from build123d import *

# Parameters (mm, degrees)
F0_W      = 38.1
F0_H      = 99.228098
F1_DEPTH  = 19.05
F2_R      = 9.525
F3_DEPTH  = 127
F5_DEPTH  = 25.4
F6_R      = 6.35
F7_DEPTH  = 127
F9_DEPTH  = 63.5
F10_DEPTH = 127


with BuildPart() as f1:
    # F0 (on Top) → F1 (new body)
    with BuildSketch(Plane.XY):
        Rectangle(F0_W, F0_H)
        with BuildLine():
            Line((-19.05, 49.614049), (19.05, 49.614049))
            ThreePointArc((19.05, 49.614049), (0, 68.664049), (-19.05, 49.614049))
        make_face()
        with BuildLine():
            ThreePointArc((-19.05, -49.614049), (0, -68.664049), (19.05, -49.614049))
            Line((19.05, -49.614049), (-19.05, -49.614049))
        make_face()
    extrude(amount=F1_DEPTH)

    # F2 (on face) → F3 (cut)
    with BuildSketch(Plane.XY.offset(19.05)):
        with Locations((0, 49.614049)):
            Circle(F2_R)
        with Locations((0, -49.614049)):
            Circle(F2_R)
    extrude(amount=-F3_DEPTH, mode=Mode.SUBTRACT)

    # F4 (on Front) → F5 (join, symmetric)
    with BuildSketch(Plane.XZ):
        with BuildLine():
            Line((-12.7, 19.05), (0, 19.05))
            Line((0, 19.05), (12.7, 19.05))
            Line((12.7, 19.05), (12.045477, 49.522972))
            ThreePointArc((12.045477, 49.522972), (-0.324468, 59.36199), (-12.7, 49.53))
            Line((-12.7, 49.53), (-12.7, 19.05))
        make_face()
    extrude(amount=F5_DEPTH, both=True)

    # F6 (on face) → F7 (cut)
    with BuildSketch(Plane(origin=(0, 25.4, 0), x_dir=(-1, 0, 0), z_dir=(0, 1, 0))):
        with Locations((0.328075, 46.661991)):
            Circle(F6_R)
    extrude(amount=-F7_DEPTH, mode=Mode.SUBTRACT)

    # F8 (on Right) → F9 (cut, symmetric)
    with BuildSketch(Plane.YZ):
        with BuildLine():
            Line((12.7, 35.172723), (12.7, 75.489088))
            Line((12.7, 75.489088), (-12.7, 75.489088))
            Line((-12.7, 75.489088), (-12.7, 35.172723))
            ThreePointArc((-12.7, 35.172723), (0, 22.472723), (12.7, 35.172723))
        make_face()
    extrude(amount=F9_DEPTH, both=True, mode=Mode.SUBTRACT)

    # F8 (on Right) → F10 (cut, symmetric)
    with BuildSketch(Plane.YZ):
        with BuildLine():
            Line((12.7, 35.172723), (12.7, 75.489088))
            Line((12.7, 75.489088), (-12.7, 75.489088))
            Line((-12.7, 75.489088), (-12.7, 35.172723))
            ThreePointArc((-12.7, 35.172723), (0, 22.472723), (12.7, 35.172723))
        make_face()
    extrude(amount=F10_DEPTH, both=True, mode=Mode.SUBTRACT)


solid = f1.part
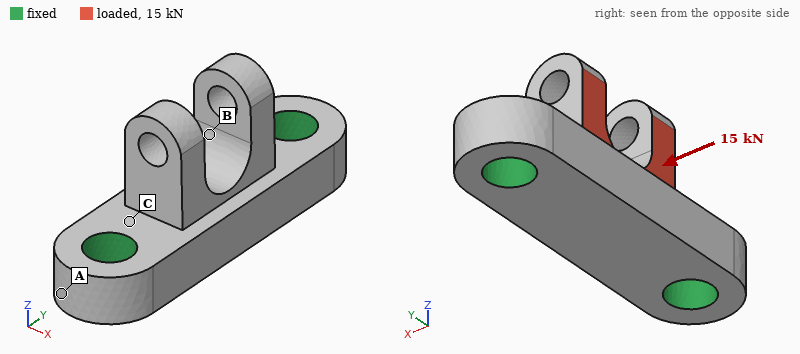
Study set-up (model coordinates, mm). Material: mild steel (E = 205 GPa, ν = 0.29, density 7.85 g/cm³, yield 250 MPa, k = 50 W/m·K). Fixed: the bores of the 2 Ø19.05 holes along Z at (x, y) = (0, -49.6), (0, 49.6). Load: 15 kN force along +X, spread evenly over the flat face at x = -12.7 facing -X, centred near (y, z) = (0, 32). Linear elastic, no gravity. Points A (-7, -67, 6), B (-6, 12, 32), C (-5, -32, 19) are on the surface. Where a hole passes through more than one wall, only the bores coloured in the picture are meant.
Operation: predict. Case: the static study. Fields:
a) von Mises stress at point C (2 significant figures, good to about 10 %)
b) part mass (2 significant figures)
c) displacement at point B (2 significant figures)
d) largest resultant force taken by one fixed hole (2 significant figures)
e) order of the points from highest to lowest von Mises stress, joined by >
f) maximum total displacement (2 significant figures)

89 MPa
840 g
27 µm
7.5 kN
C > B > A
58 µm
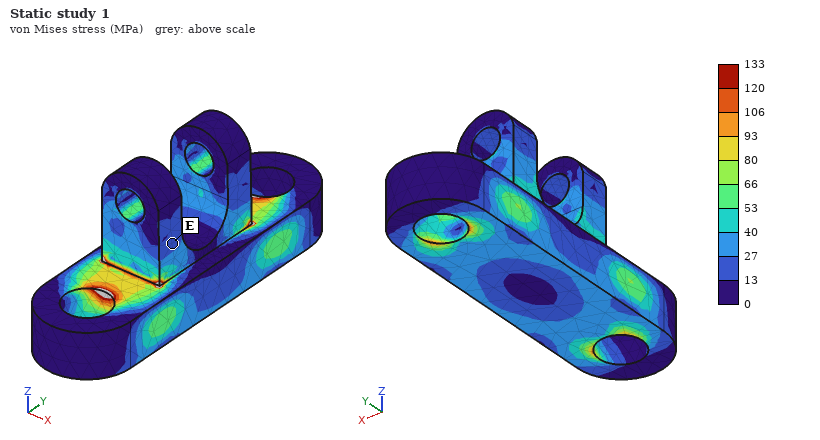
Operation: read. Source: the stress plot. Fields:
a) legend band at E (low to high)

13 to 27 MPa
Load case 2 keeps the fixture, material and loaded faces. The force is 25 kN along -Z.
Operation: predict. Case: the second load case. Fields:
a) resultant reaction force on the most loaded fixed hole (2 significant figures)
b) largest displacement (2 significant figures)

13 kN
61 µm
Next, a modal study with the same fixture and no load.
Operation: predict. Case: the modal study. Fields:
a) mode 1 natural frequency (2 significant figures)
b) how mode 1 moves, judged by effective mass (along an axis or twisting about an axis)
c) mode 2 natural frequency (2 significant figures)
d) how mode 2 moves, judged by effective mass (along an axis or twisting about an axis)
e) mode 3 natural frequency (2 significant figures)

6300 Hz
along X
7500 Hz
along Z
8300 Hz
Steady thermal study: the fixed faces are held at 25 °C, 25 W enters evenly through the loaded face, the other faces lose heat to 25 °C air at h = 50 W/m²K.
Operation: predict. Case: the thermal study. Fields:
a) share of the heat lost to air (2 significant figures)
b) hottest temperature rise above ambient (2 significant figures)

24 %
20 K
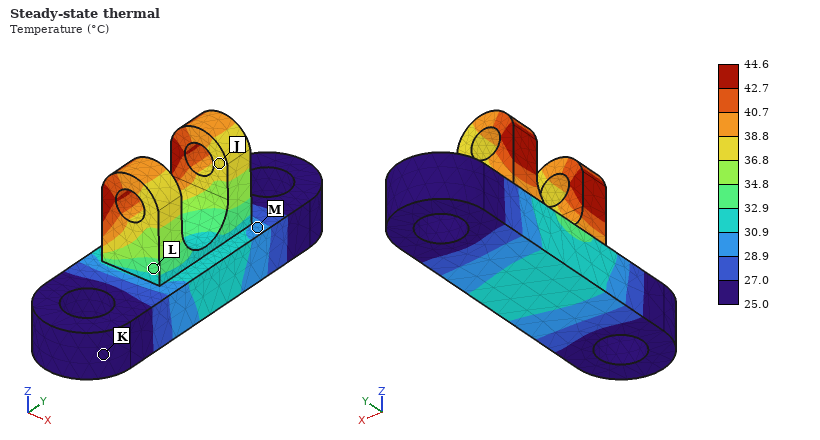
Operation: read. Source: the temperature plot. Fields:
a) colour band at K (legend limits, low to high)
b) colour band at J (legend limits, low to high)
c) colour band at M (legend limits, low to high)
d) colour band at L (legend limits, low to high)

25.0 to 27.0 °C
36.8 to 38.8 °C
28.9 to 30.9 °C
32.9 to 34.8 °C
